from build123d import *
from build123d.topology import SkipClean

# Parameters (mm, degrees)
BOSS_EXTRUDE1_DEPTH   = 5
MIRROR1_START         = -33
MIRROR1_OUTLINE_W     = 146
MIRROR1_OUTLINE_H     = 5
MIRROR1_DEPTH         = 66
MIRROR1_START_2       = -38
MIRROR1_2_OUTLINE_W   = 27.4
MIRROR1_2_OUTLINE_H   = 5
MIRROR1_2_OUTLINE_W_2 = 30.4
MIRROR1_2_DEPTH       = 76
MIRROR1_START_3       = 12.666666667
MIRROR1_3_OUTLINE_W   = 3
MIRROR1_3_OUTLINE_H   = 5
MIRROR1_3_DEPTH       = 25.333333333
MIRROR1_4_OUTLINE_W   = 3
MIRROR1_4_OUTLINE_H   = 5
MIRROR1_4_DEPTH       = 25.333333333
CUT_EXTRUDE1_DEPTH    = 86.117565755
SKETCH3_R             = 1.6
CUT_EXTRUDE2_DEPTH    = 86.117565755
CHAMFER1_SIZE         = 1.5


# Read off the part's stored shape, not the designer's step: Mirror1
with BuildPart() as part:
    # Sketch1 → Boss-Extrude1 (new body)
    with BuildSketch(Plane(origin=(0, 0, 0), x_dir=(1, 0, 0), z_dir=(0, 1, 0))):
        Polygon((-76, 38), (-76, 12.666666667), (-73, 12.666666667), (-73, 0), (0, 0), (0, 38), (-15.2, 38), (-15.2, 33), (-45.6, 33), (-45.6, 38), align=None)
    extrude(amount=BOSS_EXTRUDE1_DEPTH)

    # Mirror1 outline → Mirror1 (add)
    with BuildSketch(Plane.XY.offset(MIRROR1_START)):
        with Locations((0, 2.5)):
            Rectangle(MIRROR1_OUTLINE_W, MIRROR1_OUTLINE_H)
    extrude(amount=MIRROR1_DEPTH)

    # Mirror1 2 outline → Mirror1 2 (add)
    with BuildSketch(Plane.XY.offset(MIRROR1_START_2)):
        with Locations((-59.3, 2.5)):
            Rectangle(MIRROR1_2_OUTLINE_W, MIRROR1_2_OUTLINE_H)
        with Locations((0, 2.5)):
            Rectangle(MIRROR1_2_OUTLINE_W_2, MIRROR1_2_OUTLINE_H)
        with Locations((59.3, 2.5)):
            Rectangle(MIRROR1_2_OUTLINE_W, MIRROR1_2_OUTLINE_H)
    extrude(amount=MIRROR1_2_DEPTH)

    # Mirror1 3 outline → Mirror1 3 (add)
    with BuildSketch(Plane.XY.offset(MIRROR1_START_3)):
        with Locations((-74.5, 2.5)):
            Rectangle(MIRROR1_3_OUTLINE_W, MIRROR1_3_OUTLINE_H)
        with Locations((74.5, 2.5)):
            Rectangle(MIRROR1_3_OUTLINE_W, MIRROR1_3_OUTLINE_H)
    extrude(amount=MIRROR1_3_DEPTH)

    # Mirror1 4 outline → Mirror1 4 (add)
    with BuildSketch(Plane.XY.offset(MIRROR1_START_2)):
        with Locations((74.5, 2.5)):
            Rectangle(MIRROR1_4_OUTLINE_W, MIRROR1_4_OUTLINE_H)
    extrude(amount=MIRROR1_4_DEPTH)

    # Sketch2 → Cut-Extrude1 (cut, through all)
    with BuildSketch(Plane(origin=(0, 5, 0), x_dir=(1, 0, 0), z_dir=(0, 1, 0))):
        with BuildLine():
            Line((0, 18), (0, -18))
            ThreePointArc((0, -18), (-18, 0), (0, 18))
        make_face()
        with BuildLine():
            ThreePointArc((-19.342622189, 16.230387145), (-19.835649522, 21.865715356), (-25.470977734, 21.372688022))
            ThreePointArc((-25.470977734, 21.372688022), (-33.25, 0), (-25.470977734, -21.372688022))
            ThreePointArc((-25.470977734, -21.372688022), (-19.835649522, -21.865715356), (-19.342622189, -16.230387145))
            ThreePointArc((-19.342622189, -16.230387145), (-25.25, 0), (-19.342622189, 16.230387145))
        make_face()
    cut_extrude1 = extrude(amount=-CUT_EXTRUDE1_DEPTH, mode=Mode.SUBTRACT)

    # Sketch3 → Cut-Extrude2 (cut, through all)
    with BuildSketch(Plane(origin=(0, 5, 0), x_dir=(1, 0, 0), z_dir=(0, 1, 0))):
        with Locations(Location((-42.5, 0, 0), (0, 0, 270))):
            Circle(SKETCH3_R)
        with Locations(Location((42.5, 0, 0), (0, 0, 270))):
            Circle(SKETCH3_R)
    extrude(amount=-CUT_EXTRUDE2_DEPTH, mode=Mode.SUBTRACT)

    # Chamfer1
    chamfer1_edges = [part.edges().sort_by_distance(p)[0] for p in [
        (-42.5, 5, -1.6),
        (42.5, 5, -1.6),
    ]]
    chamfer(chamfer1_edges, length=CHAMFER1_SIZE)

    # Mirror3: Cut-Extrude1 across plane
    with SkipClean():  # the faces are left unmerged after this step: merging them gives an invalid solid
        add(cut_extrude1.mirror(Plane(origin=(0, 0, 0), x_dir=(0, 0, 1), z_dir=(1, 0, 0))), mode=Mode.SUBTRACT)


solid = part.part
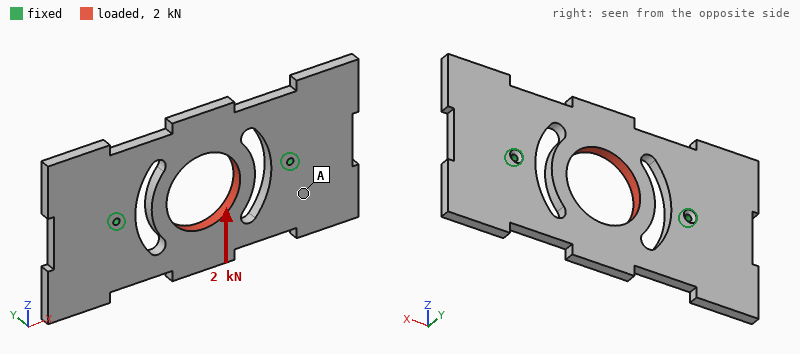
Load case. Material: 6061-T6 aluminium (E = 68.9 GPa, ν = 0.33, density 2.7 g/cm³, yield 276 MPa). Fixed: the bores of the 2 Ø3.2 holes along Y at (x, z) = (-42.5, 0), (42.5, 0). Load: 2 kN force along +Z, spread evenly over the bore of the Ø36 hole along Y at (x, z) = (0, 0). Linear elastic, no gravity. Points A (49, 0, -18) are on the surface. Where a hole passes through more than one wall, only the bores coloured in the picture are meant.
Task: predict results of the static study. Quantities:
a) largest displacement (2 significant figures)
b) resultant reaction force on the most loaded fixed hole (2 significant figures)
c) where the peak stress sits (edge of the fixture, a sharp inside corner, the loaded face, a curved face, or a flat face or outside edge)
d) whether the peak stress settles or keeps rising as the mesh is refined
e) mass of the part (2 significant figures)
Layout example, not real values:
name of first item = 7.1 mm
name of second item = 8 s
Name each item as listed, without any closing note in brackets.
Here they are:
largest displacement = 23 µm
resultant reaction force on the most loaded fixed hole = 1.0 kN
where the peak stress sits = edge of the fixture
whether the peak stress settles or keeps rising as the mesh is refined = keeps rising
mass of the part = 120 g
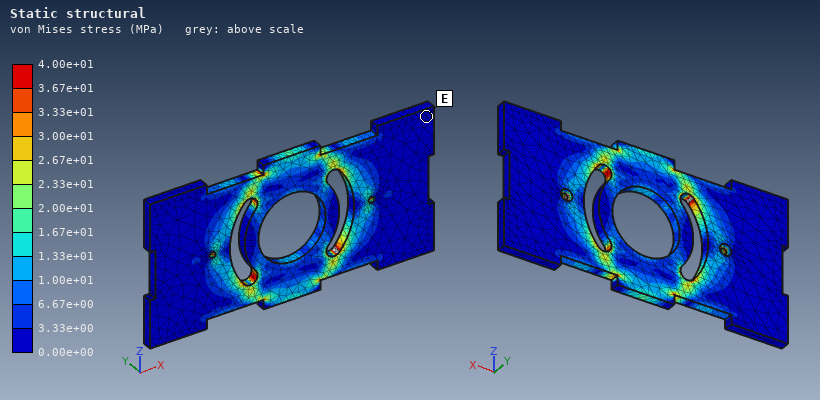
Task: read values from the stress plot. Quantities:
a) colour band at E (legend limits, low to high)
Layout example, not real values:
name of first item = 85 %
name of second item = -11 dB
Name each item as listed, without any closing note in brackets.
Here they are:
colour band at E = 0.00e+00 to 3.33e+00 MPa
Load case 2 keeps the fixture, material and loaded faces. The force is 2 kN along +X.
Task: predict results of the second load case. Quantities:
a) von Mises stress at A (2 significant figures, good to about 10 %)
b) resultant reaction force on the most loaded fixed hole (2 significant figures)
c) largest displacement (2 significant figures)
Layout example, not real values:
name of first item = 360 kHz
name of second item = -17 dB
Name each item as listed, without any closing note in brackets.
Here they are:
von Mises stress at A = 6.1 MPa
resultant reaction force on the most loaded fixed hole = 1.0 kN
largest displacement = 17 µm
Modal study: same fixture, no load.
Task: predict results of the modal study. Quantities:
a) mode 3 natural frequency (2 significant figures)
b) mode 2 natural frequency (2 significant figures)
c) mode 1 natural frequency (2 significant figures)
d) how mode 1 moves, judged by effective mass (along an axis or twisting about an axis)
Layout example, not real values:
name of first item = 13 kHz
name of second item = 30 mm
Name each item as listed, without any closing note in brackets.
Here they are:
mode 3 natural frequency = 1700 Hz
mode 2 natural frequency = 1600 Hz
mode 1 natural frequency = 1200 Hz
how mode 1 moves, judged by effective mass = twisting about X
